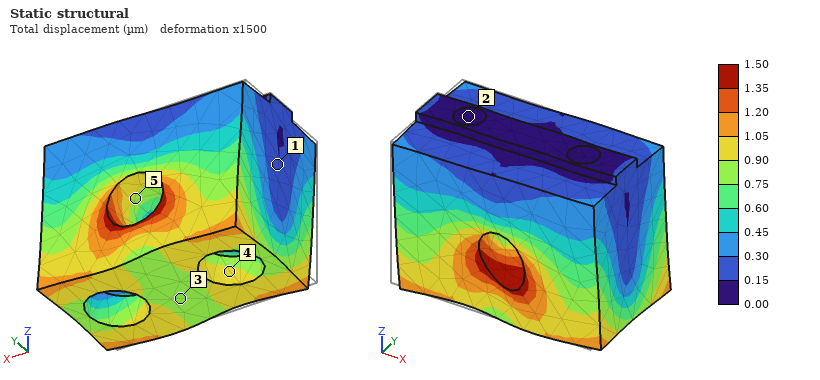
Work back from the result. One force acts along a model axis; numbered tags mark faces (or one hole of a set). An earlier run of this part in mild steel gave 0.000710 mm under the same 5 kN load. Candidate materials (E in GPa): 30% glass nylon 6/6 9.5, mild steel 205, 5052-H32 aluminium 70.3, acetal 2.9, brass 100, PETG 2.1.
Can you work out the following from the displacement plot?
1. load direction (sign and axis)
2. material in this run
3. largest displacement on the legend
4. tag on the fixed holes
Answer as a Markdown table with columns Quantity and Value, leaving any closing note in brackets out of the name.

| Quantity | Value |
|---|---|
| load direction | +X |
| material in this run | brass |
| largest displacement on the legend | 1.50 µm |
| tag on the fixed holes | 2 |
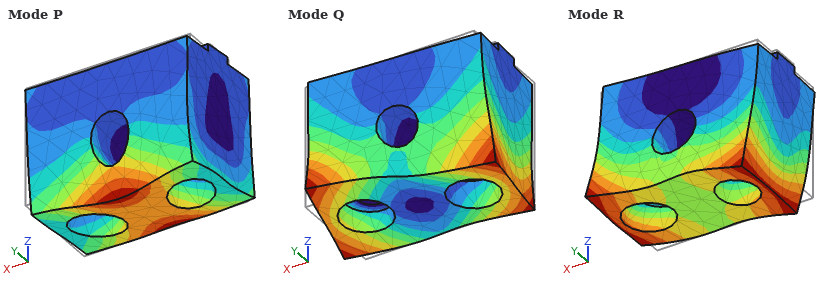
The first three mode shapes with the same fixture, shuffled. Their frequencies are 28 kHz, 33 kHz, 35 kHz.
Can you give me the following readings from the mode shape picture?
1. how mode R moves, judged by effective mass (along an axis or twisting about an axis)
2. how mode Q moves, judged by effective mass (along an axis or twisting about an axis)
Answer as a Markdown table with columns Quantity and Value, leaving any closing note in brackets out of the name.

| Quantity | Value |
|---|---|
| how mode R moves, judged by effective mass | along X |
| how mode Q moves, judged by effective mass | twisting about Z |
